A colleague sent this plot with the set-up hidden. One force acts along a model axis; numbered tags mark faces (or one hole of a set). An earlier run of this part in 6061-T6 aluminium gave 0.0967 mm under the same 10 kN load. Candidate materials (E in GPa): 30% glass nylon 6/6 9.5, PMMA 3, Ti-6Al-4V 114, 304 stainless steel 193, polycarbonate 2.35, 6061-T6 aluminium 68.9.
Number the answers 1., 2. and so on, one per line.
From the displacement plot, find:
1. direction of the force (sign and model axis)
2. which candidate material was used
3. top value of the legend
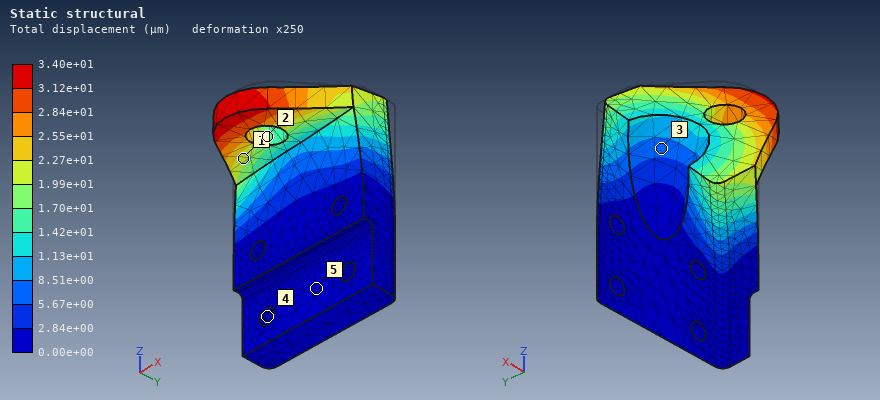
1. -X
2. 304 stainless steel
3. 3.40e+01 µm
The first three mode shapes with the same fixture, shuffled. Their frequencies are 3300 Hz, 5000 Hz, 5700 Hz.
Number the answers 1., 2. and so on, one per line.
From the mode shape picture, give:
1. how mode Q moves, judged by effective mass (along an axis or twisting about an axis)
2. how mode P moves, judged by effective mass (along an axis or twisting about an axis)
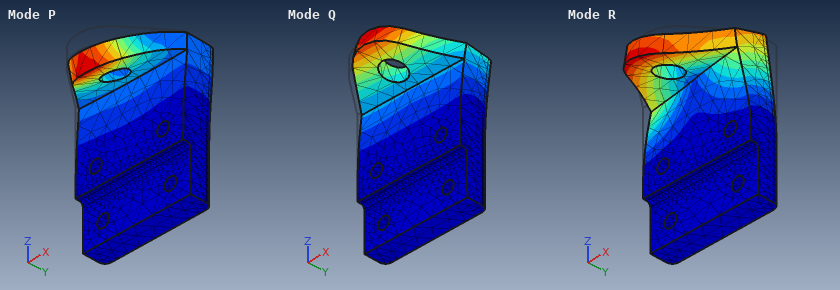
1. along Y
2. along Y
